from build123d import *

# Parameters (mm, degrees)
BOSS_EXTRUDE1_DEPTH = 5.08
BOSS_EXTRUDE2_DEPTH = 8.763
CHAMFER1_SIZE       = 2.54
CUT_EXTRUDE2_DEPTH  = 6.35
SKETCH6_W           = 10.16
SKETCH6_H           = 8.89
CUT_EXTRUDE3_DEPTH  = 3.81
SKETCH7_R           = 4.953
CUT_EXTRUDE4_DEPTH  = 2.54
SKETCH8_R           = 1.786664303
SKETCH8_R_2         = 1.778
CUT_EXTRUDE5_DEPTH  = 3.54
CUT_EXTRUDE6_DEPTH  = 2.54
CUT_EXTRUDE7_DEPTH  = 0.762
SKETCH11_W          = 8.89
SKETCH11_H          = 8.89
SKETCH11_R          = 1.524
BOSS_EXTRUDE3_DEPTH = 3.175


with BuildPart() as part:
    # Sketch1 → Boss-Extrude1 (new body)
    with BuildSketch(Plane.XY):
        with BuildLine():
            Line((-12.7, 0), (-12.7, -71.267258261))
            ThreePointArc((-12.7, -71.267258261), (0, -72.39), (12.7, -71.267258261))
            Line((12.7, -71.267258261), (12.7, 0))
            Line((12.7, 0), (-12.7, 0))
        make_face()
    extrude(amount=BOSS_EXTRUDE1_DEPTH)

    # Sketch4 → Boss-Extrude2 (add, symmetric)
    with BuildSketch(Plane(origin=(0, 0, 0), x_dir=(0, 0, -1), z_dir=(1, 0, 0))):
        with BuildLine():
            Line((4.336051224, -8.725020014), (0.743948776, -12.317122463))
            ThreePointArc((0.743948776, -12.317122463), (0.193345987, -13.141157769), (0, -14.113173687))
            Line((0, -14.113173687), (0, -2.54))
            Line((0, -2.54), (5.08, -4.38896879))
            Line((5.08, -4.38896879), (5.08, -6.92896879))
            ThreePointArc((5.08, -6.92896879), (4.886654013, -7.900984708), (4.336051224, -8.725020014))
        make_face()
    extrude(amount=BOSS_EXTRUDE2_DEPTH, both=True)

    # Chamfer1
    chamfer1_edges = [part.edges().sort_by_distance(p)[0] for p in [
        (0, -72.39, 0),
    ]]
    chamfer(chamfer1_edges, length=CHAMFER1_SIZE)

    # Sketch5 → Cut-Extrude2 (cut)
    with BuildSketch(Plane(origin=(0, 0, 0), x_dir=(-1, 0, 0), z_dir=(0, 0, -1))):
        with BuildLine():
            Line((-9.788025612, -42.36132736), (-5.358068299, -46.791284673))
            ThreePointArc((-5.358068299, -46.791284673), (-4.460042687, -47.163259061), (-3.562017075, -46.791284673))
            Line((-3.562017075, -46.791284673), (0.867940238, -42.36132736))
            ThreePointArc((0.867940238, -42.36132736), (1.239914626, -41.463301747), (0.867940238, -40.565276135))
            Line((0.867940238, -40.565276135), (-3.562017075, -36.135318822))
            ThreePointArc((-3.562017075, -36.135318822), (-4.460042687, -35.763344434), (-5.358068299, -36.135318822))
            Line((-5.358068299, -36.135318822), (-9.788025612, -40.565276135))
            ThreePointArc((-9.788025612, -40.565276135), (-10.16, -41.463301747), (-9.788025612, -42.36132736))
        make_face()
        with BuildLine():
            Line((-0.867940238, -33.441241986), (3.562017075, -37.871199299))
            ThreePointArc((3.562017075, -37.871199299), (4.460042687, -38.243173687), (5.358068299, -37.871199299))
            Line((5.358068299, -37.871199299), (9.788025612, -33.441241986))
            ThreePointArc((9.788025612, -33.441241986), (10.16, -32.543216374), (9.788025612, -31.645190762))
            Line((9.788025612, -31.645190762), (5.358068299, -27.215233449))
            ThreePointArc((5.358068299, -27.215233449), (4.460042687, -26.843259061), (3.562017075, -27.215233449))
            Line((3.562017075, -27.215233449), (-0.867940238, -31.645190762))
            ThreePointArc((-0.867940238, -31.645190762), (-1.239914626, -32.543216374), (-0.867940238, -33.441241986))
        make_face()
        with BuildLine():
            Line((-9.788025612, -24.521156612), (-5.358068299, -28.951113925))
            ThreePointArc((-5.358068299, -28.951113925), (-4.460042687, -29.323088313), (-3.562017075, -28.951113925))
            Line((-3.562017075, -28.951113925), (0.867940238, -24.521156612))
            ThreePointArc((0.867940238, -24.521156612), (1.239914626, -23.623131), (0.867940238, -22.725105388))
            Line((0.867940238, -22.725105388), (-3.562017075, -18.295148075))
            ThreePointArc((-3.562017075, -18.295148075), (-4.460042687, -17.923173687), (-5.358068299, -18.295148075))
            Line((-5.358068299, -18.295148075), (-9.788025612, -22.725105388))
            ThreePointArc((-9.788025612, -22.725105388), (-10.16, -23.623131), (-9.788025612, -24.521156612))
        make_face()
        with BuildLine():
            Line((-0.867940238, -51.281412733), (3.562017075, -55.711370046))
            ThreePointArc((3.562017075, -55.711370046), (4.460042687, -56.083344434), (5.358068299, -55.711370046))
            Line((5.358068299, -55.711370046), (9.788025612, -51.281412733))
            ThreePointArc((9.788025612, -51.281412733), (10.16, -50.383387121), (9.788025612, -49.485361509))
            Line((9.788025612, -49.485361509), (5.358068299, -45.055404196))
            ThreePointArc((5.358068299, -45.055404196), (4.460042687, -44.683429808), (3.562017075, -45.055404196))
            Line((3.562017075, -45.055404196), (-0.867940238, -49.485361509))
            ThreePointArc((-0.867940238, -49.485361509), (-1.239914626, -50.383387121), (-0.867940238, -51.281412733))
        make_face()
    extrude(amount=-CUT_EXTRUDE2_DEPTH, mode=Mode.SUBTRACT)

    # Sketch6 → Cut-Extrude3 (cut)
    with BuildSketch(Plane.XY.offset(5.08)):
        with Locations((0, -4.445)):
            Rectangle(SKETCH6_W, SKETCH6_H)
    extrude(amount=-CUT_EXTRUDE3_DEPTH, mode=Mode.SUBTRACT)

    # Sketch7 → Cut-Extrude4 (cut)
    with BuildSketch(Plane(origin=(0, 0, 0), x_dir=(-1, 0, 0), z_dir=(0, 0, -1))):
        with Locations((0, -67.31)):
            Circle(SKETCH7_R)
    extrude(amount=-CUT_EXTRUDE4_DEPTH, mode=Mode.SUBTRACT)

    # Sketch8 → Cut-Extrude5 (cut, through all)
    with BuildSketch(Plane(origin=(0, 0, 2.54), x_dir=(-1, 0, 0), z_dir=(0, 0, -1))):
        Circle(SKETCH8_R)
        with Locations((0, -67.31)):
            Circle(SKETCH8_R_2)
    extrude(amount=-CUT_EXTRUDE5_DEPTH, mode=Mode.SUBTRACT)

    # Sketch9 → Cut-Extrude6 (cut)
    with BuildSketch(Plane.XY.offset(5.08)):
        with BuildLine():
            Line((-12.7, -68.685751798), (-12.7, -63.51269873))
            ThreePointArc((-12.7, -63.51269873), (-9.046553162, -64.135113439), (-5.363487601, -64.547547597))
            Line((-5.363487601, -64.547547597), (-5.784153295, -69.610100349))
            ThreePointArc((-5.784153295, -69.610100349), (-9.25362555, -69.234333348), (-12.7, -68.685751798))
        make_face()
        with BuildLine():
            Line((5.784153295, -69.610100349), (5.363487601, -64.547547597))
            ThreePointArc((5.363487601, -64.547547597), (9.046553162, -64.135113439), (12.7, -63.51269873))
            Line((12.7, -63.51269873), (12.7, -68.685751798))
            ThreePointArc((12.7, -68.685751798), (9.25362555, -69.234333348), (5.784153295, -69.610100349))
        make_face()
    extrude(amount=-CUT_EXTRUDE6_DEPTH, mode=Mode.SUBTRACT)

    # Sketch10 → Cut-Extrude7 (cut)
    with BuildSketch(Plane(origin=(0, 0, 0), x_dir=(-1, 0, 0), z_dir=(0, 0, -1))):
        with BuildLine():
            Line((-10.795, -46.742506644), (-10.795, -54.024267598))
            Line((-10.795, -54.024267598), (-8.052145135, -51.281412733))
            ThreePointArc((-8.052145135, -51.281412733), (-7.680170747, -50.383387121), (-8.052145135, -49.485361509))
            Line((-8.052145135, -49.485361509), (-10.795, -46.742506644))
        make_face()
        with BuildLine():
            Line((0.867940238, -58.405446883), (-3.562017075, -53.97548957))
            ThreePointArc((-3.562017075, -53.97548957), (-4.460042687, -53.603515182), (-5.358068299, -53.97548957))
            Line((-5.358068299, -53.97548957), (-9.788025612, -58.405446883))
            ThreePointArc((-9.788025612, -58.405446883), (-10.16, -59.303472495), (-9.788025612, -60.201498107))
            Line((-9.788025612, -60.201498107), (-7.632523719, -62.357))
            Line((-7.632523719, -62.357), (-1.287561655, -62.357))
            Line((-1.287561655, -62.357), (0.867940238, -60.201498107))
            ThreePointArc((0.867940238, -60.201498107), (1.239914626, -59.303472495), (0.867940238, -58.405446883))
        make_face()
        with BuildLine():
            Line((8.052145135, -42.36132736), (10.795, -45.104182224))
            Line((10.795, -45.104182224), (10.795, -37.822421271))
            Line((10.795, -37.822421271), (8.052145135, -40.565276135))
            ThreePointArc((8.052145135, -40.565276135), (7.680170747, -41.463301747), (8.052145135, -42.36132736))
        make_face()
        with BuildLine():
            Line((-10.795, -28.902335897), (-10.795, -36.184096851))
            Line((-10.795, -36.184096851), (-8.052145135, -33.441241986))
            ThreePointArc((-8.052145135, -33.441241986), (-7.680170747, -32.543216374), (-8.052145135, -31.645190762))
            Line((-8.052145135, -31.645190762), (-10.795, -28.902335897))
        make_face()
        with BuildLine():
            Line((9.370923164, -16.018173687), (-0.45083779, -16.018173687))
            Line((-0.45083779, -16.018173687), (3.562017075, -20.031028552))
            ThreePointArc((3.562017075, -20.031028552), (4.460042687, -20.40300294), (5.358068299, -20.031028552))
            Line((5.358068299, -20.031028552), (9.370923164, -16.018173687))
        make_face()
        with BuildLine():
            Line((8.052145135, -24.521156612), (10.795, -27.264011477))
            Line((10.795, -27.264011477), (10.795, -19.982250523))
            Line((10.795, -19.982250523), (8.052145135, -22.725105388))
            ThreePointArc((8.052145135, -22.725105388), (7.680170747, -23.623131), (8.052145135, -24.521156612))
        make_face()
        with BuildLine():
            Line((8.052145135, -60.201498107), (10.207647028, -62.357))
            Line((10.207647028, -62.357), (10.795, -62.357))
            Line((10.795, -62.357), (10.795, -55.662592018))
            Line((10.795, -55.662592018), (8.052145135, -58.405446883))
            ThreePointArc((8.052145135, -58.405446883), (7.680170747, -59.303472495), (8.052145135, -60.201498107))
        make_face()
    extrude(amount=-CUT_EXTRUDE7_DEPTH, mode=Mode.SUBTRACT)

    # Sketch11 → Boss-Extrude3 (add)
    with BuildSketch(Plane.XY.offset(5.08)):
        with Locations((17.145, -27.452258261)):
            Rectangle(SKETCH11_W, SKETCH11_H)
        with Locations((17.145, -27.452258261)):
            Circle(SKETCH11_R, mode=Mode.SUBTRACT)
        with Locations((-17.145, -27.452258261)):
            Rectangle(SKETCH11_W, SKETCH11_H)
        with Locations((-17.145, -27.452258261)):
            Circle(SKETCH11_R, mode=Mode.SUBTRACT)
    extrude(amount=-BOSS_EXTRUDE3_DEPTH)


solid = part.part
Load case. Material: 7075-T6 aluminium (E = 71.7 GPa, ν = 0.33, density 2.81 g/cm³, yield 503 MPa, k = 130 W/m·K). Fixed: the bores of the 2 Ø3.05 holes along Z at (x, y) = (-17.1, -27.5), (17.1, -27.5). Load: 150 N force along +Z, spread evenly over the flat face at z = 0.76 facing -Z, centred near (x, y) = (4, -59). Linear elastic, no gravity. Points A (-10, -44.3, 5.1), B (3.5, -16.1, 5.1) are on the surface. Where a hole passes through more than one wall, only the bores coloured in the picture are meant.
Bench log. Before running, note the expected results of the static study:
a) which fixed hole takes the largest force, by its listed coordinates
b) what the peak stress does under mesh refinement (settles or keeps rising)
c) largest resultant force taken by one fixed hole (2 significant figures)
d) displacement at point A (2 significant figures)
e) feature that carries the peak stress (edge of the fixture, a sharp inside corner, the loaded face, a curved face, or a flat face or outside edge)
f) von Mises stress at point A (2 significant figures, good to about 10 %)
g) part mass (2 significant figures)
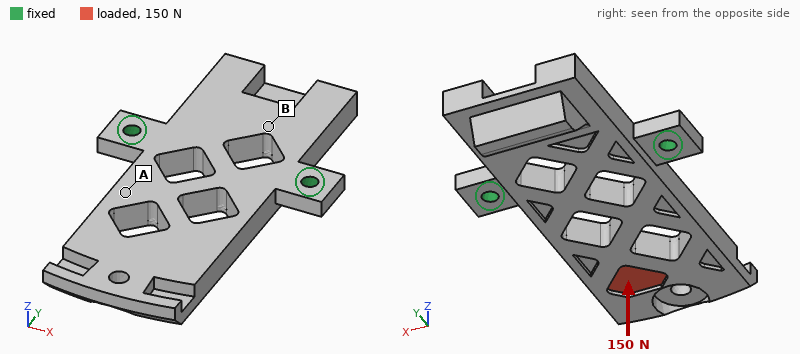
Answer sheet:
(17.1, -27.5)
keeps rising
120 N
0.13 mm
edge of the fixture
34 MPa
22 g
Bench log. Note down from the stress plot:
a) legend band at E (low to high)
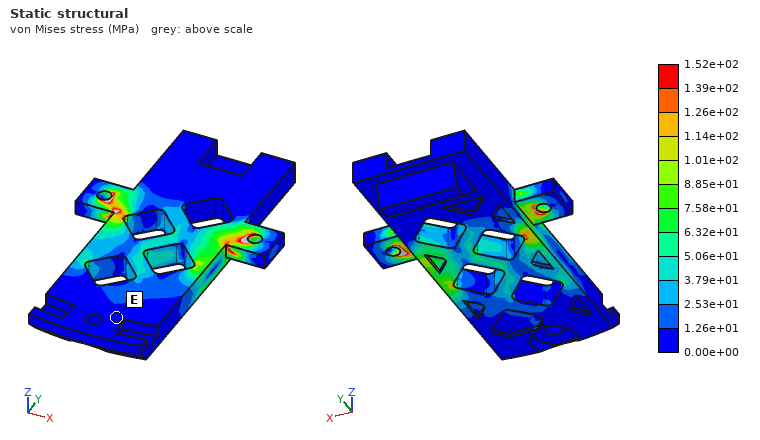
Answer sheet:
0.00e+00 to 1.26e+01 MPa
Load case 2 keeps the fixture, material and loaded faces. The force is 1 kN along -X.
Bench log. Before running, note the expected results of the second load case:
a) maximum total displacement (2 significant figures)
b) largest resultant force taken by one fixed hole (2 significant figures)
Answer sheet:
0.11 mm
1.2 kN
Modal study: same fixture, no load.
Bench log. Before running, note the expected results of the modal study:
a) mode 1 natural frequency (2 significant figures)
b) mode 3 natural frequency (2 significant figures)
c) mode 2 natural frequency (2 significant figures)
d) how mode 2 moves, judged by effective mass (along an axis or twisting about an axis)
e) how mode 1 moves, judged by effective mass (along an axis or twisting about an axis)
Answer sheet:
1200 Hz
5700 Hz
2800 Hz
along Z
along Z
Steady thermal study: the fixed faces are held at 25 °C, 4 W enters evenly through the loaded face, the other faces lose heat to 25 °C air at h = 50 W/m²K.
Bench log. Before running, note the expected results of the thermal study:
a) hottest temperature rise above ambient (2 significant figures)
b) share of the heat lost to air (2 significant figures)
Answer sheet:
13 K
36 %
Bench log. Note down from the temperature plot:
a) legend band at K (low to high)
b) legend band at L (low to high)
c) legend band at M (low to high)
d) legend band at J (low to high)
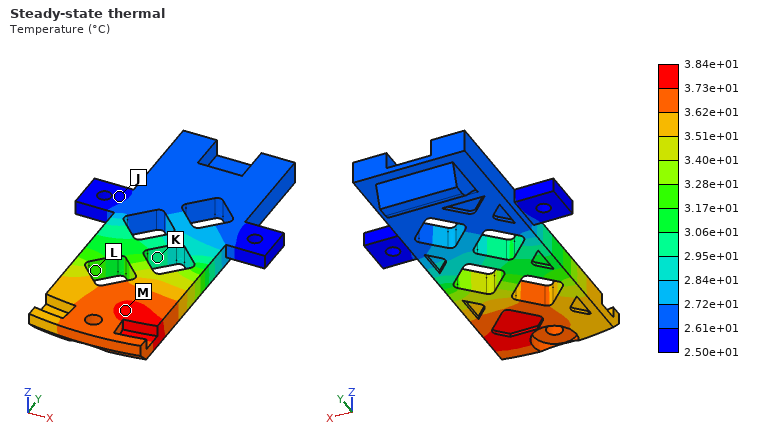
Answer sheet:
2.95e+01 to 3.06e+01 °C
3.17e+01 to 3.28e+01 °C
3.73e+01 to 3.84e+01 °C
2.50e+01 to 2.61e+01 °C
